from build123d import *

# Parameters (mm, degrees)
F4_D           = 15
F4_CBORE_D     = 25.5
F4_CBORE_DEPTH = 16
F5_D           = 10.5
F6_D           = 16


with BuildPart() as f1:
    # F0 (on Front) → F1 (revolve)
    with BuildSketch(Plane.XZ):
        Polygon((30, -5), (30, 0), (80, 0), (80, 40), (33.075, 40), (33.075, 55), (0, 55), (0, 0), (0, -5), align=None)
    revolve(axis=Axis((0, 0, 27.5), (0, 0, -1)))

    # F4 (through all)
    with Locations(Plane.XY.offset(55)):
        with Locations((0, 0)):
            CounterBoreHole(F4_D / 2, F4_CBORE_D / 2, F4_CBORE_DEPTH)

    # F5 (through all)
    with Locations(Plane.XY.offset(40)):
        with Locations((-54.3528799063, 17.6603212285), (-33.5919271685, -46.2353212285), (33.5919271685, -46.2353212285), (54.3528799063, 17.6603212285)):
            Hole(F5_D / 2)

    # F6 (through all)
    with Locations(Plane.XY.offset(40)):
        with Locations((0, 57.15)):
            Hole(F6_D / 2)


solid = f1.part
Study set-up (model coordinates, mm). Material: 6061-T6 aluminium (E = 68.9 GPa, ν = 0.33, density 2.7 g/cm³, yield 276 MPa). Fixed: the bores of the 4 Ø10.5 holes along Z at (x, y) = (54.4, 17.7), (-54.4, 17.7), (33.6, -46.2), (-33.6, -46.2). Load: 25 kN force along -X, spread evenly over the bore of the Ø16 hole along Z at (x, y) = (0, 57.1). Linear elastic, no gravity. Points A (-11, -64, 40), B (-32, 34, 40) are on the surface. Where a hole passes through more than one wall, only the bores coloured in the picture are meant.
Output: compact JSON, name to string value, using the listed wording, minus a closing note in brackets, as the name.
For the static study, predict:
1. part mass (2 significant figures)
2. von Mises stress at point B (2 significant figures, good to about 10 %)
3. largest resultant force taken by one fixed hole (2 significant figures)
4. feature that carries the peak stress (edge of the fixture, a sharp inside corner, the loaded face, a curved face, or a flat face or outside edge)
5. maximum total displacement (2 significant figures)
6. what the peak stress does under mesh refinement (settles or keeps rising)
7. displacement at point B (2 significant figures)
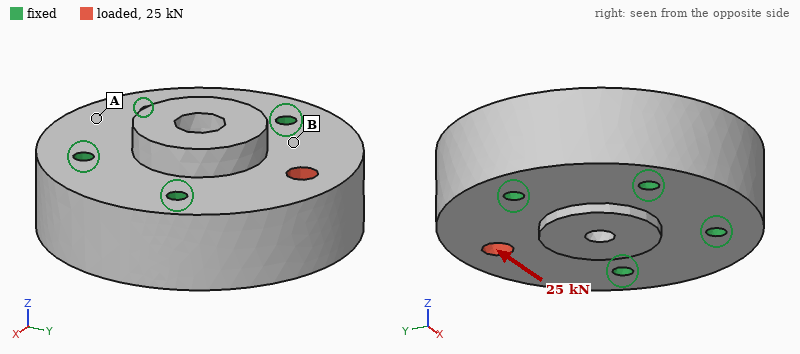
{"part mass": "2.2 kg", "von Mises stress at point B": "9.2 MPa", "largest resultant force taken by one fixed hole": "14 kN", "feature that carries the peak stress": "edge of the fixture", "maximum total displacement": "14 µm", "what the peak stress does under mesh refinement": "keeps rising", "displacement at point B": "4.2 µm"}
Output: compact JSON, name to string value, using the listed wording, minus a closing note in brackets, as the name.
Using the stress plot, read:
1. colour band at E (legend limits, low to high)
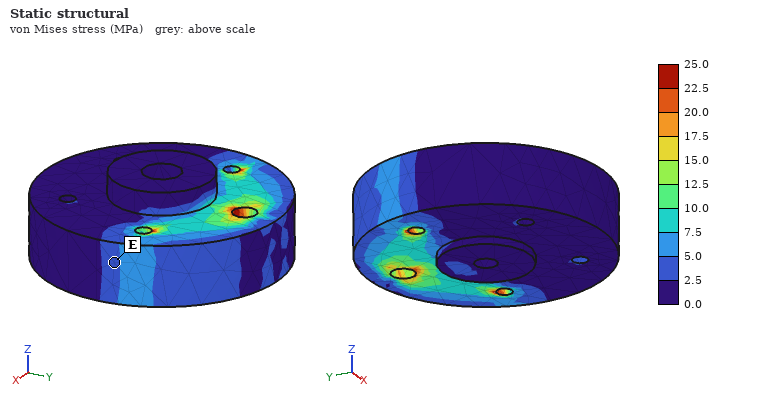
{"colour band at E": "2.5 to 5.0 MPa"}
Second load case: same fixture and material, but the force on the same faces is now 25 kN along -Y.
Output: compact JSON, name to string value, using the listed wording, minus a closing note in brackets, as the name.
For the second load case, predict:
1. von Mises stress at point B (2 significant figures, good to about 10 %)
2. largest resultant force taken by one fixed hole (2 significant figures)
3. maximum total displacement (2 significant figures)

{"von Mises stress at point B": "6.9 MPa", "largest resultant force taken by one fixed hole": "8.4 kN", "maximum total displacement": "13 µm"}
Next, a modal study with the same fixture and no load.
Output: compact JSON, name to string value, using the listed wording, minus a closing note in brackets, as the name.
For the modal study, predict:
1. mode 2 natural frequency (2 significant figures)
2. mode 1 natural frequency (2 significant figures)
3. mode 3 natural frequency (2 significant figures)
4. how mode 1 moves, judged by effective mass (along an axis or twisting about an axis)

{"mode 2 natural frequency": "12 kHz", "mode 1 natural frequency": "6100 Hz", "mode 3 natural frequency": "12 kHz", "how mode 1 moves, judged by effective mass": "along Z"}
